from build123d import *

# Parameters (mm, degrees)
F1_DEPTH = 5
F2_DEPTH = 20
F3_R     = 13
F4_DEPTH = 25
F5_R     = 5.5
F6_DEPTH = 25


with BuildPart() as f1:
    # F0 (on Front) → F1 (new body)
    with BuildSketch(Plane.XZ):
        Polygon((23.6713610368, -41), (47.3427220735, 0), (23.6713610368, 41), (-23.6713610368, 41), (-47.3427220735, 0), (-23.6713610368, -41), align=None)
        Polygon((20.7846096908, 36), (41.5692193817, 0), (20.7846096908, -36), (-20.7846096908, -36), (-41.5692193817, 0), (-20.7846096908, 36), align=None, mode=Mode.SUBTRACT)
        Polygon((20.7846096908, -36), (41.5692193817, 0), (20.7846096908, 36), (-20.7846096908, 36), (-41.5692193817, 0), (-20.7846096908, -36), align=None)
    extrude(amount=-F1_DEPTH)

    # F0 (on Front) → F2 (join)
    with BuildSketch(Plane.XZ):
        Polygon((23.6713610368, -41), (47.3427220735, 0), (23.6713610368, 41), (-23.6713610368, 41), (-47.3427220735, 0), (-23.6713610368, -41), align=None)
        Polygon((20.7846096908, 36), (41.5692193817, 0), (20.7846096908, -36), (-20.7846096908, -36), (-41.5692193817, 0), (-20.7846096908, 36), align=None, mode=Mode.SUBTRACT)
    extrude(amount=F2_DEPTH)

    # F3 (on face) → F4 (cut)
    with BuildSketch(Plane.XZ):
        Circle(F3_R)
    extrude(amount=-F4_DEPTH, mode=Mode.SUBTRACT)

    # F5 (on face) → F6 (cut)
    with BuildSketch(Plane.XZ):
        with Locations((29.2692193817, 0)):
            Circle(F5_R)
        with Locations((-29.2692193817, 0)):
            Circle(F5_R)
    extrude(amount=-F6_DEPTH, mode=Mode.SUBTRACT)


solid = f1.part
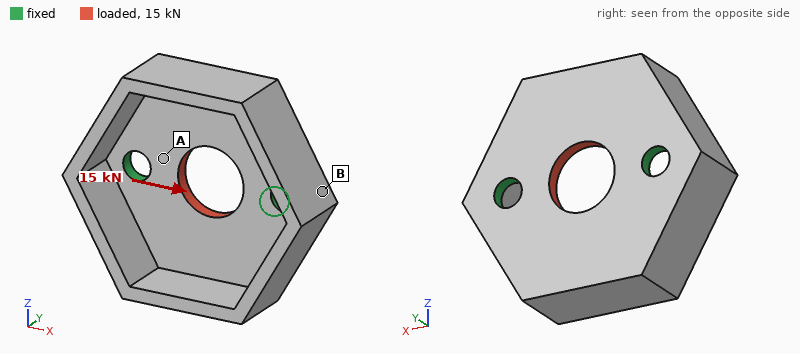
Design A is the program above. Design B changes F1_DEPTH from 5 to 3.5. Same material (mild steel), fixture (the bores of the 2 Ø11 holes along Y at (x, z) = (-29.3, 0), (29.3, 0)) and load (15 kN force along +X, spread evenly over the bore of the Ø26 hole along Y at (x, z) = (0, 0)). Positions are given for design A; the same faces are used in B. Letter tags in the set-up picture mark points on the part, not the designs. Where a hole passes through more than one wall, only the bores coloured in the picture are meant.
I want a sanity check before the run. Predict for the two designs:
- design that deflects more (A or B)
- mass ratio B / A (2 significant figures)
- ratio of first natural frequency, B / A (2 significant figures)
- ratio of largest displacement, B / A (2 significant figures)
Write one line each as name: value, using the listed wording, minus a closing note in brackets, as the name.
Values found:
design that deflects more: B
mass ratio B / A: 0.85
ratio of first natural frequency, B / A: 0.73
ratio of largest displacement, B / A: 1.4
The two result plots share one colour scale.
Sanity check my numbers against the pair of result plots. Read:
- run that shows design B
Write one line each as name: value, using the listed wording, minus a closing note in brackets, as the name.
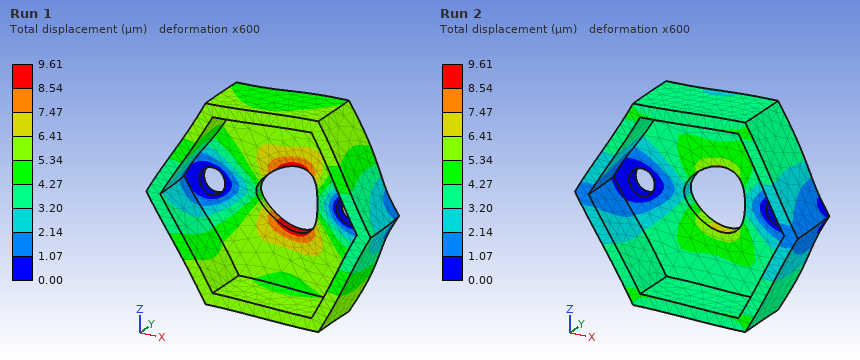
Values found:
run that shows design B: Run 1
